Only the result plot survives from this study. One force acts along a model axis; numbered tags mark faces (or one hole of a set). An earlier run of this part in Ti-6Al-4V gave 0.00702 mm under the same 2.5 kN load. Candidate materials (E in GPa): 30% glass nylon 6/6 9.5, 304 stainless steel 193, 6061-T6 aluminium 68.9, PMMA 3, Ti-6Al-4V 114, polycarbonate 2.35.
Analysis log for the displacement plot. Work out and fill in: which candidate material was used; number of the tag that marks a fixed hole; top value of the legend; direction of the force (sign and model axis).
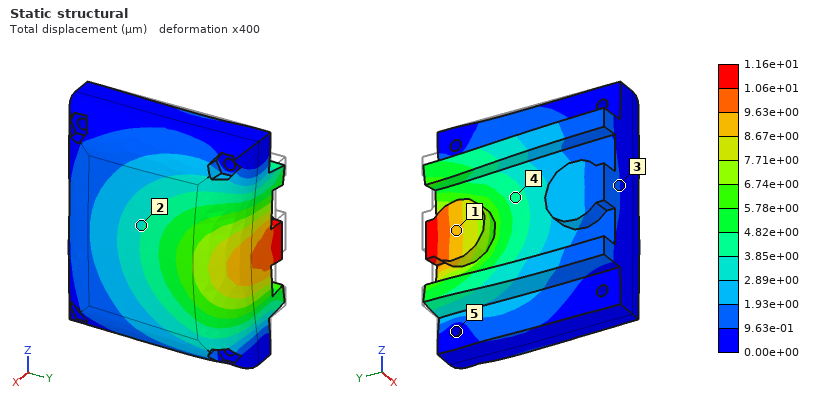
6061-T6 aluminium
5
1.16e+01 µm
+X
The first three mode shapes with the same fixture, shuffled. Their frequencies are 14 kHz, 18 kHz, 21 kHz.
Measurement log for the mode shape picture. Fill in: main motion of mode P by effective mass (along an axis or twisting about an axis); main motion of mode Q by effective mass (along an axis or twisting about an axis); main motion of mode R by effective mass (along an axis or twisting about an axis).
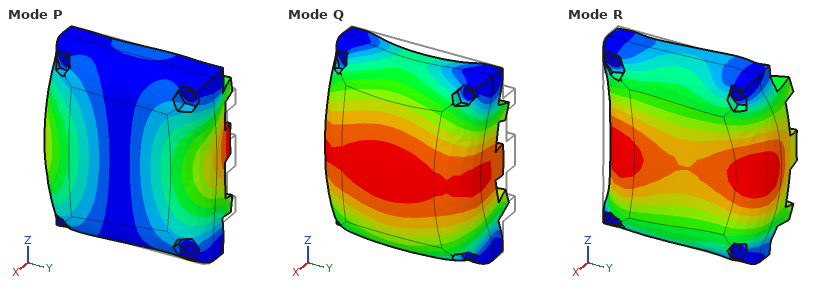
along Y
along X
along Y
